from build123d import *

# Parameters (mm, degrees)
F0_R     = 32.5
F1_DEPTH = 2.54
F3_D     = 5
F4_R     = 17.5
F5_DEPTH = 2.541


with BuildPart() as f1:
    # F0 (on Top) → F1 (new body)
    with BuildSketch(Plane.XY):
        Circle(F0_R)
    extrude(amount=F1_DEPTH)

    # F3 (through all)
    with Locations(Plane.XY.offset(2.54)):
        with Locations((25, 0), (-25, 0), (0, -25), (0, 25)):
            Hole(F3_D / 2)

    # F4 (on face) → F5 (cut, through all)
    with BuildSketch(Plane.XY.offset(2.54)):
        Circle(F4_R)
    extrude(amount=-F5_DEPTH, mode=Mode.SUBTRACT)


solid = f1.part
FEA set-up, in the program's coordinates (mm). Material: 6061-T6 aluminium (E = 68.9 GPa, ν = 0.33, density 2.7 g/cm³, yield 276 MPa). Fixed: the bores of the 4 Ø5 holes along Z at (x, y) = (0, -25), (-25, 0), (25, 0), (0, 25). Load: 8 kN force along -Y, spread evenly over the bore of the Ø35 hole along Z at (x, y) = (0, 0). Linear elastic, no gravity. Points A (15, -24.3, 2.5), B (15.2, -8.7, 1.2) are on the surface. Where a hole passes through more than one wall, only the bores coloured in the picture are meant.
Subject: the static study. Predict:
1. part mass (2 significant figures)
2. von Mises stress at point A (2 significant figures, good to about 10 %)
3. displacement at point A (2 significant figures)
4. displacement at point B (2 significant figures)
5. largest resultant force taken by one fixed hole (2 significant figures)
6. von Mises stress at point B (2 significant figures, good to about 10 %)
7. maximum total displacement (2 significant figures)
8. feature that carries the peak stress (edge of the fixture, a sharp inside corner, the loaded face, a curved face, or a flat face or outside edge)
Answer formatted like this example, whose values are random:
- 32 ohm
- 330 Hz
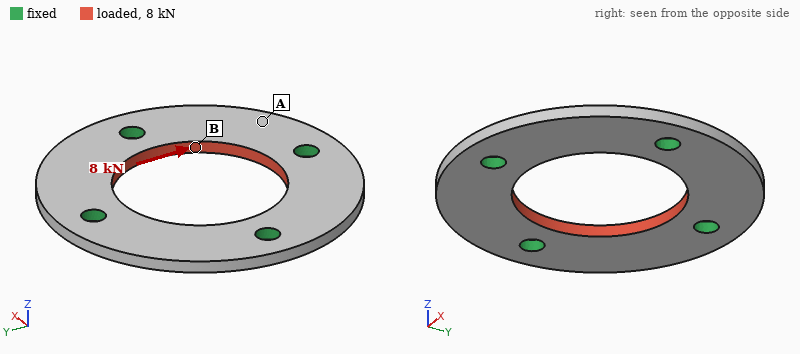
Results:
- 16 g
- 20 MPa
- 10 µm
- 13 µm
- 2.2 kN
- 45 MPa
- 14 µm
- edge of the fixture
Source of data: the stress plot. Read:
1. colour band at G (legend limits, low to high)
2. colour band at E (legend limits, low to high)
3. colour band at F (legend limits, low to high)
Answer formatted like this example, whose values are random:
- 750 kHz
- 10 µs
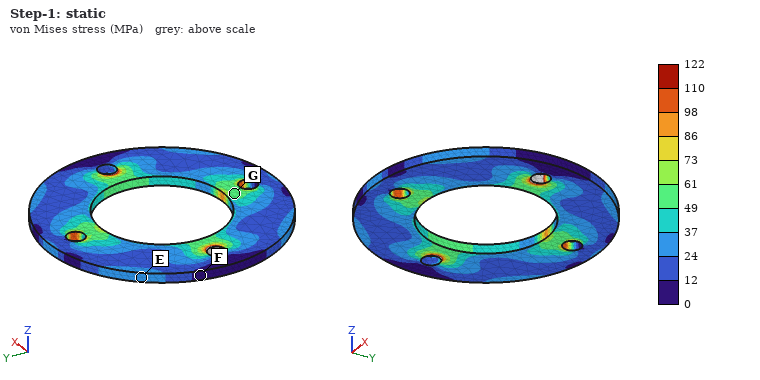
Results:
- 49 to 61 MPa
- 24 to 37 MPa
- 0 to 12 MPa
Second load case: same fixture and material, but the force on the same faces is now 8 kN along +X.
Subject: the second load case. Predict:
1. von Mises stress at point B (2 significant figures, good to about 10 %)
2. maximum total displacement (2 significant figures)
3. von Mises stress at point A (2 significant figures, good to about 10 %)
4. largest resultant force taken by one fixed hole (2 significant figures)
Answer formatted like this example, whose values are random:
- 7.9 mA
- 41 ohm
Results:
- 37 MPa
- 14 µm
- 23 MPa
- 2.2 kN
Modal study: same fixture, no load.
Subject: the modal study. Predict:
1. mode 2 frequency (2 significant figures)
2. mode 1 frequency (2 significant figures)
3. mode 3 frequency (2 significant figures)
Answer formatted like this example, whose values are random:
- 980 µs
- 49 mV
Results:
- 8000 Hz
- 8000 Hz
- 8000 Hz
